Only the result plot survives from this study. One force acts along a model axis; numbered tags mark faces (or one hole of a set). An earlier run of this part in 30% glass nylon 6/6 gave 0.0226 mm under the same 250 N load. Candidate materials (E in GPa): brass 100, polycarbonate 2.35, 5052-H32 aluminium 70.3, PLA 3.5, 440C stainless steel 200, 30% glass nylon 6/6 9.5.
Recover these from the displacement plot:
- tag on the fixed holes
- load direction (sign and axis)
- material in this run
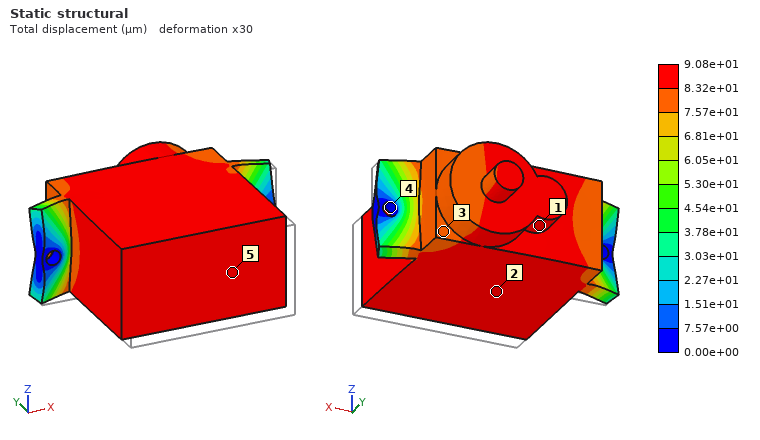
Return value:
4
+Y
polycarbonate
